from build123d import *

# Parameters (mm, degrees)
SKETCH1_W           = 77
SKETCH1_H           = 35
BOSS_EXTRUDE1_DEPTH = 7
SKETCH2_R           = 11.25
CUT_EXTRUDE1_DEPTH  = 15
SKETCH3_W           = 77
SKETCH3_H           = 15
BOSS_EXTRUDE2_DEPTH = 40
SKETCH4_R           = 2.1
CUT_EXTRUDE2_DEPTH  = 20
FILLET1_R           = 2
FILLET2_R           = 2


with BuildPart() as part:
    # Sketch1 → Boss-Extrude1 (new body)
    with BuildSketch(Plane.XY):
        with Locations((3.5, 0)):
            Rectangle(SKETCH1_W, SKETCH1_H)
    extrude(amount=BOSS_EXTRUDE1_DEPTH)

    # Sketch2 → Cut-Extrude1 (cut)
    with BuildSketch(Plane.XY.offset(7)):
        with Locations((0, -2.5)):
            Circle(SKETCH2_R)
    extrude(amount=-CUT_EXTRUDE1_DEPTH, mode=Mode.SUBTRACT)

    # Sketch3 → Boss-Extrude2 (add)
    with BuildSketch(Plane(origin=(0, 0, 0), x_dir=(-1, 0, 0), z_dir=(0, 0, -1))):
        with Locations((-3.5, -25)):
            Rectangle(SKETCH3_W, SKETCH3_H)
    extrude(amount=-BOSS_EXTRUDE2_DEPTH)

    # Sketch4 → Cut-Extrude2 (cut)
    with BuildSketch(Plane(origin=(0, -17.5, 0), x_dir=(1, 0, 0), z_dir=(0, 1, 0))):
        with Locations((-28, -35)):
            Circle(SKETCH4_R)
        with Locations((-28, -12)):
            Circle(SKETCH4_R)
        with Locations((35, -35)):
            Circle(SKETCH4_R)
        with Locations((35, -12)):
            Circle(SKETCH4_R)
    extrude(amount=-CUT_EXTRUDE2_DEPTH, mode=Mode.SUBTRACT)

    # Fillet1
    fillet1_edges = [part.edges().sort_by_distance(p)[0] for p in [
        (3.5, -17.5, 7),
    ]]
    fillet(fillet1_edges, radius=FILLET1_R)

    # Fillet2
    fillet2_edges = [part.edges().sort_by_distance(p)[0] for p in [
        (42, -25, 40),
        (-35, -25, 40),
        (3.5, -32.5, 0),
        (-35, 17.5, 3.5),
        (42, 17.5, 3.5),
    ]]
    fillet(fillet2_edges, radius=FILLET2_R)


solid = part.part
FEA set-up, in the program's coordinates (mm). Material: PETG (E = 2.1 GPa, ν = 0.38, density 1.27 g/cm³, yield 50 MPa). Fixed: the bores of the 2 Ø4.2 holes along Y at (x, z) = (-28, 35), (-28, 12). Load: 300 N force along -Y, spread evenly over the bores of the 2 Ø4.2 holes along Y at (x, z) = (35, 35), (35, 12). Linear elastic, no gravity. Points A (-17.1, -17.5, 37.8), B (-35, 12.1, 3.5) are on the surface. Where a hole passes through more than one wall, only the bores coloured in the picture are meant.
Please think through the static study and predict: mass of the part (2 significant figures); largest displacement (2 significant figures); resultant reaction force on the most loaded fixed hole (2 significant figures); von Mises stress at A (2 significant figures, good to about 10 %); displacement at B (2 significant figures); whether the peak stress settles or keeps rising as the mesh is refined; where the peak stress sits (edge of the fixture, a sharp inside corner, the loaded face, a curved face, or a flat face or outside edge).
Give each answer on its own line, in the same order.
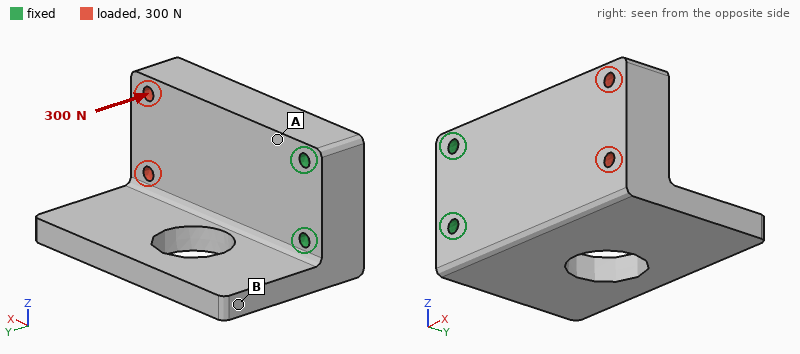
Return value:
78 g
1.1 mm
150 N
9.2 MPa
0.46 mm
keeps rising
edge of the fixture
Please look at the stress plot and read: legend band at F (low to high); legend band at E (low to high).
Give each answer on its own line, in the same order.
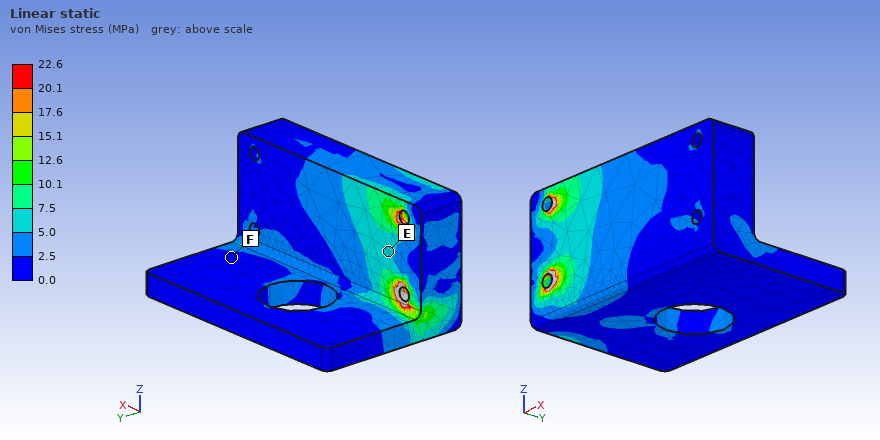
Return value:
0.0 to 2.5 MPa
5.0 to 7.5 MPa
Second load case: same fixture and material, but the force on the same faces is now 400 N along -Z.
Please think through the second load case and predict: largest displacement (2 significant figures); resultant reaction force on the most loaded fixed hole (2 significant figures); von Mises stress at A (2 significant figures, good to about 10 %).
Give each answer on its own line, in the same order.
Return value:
0.37 mm
1.0 kN
5.4 MPa
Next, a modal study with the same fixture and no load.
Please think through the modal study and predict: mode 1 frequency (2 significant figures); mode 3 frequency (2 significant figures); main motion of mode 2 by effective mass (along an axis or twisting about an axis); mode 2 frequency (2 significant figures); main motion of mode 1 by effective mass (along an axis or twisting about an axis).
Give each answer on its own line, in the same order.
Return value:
530 Hz
1100 Hz
along Z
730 Hz
along Y
